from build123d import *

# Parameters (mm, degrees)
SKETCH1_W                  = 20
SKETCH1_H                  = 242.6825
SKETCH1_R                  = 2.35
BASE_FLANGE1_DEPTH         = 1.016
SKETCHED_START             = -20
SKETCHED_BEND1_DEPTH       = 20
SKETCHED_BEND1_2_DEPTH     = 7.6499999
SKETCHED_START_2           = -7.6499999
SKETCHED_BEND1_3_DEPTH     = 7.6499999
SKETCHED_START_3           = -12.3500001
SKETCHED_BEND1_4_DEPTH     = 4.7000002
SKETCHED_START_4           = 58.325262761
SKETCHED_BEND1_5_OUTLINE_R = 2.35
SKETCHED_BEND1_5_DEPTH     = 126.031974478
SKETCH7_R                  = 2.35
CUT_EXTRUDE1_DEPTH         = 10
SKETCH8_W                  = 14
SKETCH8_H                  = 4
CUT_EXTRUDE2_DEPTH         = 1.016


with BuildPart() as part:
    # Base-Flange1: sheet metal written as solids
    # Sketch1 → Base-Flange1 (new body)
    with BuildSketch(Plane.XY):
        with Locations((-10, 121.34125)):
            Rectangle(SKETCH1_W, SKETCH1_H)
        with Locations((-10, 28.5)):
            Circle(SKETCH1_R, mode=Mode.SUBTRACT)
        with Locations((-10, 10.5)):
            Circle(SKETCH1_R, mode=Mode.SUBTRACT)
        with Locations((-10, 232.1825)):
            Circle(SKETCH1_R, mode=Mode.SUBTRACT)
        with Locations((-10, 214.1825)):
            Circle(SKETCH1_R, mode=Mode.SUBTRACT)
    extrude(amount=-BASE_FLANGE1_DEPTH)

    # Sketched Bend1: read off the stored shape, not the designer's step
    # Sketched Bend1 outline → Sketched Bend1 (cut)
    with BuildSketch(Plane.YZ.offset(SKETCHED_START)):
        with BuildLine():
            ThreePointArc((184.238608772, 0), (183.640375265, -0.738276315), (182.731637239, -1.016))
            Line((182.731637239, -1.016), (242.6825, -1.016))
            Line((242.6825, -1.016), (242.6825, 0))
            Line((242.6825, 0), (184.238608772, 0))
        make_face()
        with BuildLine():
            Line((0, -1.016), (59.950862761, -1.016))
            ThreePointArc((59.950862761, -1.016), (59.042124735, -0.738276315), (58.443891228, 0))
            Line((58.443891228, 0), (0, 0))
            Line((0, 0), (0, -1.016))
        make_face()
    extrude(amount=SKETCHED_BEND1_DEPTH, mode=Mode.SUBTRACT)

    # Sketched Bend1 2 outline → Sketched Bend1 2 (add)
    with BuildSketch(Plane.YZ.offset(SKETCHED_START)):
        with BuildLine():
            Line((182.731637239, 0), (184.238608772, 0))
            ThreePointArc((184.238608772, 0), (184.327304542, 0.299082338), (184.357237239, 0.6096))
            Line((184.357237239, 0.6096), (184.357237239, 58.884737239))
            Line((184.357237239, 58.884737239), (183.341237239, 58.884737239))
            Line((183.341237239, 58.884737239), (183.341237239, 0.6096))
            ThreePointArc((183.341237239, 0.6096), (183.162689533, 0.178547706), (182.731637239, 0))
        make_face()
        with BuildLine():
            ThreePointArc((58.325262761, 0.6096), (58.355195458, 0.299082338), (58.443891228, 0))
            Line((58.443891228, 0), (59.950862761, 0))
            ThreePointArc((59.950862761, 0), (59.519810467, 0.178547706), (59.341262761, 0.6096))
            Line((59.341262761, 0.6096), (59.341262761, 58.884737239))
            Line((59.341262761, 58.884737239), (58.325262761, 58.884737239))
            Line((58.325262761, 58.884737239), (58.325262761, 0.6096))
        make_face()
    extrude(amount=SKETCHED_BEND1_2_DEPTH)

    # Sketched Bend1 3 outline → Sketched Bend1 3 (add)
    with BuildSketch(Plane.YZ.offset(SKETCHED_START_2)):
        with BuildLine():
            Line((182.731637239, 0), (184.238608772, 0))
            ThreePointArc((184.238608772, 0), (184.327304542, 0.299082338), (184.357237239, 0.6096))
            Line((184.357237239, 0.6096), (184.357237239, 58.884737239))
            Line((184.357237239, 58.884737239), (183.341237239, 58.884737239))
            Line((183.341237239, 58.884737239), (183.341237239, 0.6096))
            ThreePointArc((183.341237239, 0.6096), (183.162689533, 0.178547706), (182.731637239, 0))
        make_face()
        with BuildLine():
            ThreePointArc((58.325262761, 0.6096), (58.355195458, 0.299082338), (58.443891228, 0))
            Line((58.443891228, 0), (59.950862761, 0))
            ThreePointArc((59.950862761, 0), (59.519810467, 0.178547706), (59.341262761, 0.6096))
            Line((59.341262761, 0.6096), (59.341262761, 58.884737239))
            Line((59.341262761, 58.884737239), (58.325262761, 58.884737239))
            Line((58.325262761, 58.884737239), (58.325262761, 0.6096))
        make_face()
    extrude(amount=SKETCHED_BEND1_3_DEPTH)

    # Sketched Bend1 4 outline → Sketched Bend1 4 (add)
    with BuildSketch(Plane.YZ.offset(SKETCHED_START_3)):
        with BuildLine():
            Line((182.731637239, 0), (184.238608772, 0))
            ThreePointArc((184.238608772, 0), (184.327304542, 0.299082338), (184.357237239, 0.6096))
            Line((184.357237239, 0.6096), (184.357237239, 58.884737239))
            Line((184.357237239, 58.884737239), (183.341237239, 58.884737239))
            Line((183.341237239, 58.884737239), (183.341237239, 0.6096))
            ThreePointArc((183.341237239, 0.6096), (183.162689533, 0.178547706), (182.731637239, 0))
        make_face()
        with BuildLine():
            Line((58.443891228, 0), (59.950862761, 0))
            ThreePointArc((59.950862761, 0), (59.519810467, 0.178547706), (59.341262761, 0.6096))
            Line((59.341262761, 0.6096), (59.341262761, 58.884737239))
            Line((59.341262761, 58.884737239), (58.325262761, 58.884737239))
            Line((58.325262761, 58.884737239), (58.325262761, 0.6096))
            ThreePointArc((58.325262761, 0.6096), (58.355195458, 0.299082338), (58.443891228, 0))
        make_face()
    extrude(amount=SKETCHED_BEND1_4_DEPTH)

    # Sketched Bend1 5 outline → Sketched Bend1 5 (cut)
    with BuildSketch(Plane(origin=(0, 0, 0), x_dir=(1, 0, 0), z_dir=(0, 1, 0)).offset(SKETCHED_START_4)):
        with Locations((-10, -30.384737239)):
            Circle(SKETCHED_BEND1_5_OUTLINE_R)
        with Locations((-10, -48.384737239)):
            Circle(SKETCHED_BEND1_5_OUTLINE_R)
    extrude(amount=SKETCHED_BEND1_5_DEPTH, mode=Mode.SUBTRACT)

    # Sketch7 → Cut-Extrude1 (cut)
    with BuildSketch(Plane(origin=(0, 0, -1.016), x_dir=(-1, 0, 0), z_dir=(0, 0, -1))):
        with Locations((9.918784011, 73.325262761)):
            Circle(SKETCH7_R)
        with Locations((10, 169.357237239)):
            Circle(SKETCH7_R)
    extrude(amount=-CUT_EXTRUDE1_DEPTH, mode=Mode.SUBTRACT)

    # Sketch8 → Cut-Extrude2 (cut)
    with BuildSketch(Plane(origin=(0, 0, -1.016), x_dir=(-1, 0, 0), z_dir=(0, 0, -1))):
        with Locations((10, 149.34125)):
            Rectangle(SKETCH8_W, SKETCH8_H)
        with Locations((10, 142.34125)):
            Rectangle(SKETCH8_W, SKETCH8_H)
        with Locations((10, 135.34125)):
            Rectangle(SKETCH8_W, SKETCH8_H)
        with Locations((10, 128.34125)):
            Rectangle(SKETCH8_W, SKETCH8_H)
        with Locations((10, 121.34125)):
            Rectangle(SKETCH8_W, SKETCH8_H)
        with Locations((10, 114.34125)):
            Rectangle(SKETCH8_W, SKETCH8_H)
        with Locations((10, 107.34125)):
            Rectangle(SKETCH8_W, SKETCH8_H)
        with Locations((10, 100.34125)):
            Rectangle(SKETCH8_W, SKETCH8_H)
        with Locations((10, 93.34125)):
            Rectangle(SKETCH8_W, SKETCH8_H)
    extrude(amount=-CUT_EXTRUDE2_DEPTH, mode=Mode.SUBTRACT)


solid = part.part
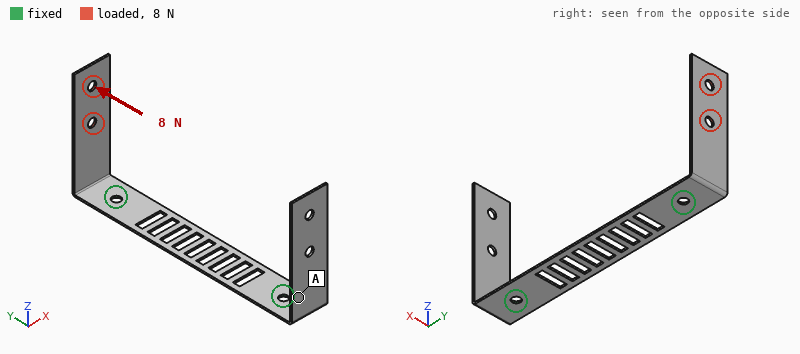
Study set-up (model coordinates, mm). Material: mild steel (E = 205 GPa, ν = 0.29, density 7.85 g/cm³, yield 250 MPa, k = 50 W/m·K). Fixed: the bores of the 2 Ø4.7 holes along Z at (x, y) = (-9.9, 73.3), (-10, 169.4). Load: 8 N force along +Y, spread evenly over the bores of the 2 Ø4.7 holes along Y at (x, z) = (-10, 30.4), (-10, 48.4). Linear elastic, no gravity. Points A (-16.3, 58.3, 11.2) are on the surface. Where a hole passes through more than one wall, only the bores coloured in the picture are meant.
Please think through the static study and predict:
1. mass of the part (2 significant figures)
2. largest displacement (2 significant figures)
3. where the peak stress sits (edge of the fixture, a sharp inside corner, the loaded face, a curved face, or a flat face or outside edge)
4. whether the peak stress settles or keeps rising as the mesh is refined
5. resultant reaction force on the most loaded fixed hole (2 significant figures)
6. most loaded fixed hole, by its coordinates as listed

34 g
1.5 mm
edge of the fixture
keeps rising
7.9 N
(-10, 169.4)
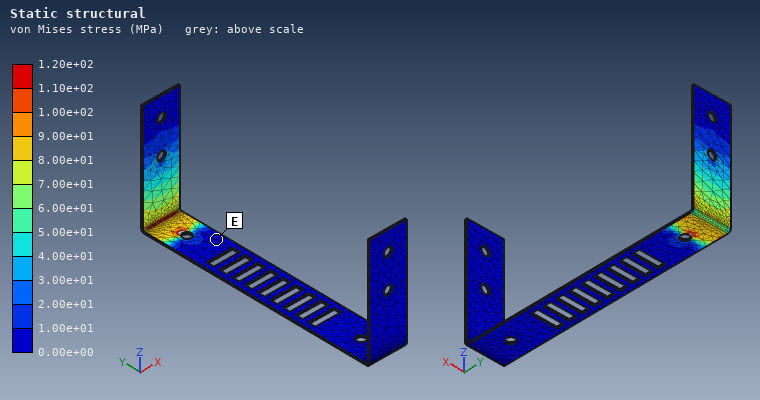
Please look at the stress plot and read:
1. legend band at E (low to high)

0.00e+00 to 1.00e+01 MPa
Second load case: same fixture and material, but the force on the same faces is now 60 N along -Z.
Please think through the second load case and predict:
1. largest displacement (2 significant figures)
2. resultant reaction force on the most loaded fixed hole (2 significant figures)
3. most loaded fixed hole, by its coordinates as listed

0.87 mm
60 N
(-10, 169.4)
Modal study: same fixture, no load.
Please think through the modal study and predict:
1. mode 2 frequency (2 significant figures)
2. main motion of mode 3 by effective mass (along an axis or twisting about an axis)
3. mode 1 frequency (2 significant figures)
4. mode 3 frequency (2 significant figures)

180 Hz
along X
180 Hz
350 Hz
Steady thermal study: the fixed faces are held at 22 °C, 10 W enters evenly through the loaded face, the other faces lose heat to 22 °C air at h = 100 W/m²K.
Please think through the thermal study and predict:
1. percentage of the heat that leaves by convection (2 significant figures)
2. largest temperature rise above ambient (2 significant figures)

96 %
72 K
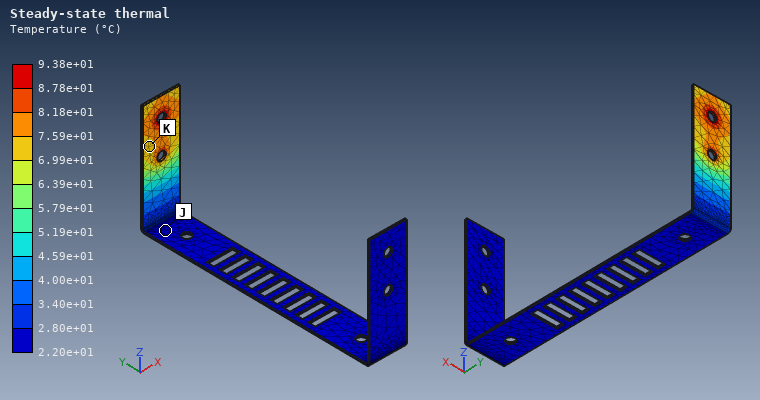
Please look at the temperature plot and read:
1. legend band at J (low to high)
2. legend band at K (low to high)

2.20e+01 to 2.80e+01 °C
6.99e+01 to 7.59e+01 °C
